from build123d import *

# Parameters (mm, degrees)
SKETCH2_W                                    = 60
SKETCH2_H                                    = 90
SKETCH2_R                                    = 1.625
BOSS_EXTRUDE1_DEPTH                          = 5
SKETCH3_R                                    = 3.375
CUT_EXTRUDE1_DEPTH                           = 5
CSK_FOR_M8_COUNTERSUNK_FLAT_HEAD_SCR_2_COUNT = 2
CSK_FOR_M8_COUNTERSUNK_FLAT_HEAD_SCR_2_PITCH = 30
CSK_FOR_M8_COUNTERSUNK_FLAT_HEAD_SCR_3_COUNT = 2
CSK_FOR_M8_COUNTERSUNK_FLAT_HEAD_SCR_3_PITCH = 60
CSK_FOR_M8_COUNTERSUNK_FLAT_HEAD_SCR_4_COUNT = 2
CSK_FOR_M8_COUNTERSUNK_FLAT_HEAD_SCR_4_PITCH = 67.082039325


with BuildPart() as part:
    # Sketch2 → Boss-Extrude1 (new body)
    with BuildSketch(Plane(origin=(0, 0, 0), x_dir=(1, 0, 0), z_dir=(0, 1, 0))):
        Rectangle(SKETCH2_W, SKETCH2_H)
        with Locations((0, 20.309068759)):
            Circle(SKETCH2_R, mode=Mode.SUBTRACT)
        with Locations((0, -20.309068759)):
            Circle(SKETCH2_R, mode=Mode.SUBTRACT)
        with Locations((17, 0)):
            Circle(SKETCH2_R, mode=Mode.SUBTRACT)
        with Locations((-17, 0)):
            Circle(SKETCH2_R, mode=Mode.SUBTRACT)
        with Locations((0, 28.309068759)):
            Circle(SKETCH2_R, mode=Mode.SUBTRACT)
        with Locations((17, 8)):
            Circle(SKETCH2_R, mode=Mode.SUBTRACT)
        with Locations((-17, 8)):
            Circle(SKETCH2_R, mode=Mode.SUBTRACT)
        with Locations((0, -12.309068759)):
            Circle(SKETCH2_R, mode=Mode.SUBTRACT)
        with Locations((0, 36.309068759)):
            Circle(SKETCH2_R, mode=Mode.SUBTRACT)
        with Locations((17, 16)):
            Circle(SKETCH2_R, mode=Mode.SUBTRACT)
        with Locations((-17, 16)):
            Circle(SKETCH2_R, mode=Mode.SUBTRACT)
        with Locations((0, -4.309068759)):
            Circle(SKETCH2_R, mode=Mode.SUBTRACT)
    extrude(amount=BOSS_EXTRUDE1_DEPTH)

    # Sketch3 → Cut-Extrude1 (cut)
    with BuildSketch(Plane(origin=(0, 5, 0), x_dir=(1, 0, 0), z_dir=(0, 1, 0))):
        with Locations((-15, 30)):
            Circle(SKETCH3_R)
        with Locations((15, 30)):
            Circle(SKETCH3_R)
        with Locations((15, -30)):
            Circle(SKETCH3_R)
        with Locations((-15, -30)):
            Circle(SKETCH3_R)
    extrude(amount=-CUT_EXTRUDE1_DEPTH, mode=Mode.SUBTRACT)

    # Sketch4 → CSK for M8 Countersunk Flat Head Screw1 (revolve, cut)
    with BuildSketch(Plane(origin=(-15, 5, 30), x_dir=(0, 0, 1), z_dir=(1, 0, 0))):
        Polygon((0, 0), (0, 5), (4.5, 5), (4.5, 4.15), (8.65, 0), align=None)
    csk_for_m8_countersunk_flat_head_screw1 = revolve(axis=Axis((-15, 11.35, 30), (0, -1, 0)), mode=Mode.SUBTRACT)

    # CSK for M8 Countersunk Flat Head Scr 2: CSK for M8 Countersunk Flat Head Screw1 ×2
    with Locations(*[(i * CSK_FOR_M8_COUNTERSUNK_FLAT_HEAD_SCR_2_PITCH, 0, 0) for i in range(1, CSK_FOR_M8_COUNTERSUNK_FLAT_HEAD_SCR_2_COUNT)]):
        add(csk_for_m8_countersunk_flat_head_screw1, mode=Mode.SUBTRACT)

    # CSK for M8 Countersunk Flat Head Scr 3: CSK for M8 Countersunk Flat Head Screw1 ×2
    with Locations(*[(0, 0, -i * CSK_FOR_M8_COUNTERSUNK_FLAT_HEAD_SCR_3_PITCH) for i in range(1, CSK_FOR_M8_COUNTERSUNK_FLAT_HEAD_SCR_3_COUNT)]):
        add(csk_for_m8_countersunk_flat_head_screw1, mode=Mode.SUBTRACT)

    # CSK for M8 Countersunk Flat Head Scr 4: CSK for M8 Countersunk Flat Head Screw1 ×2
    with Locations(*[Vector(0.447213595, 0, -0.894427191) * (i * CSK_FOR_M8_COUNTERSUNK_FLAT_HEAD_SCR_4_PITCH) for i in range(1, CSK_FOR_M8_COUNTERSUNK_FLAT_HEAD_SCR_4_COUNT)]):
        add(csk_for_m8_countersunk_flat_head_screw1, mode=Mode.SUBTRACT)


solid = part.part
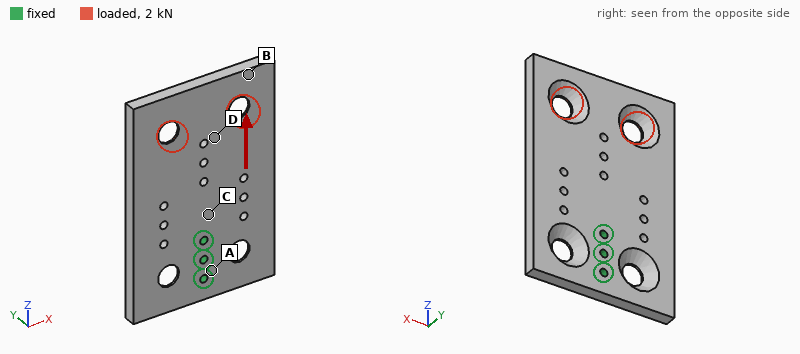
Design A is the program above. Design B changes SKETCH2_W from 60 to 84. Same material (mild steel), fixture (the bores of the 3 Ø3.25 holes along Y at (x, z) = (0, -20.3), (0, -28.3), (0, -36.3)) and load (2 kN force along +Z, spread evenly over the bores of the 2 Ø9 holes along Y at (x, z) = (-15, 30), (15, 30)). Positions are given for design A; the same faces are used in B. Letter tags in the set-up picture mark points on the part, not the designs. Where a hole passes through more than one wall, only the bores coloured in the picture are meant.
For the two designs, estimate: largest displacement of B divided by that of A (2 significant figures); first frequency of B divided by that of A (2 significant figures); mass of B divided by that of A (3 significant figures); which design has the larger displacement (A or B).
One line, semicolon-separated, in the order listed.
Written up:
0.78; 0.90; 1.45; A
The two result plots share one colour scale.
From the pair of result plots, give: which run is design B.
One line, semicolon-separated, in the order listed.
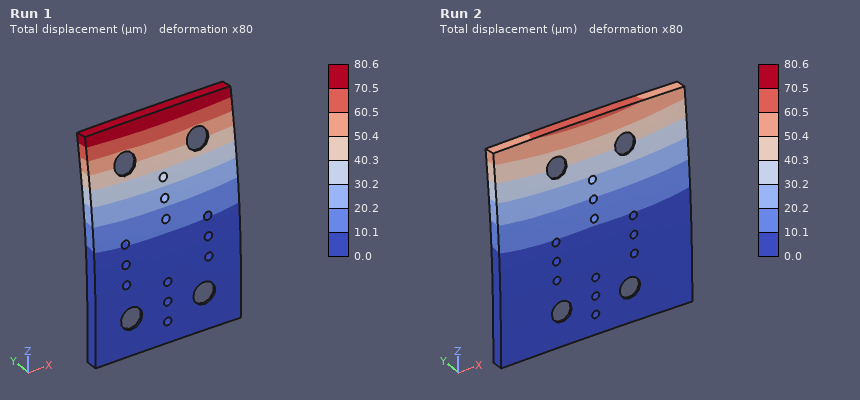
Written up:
Run 2
